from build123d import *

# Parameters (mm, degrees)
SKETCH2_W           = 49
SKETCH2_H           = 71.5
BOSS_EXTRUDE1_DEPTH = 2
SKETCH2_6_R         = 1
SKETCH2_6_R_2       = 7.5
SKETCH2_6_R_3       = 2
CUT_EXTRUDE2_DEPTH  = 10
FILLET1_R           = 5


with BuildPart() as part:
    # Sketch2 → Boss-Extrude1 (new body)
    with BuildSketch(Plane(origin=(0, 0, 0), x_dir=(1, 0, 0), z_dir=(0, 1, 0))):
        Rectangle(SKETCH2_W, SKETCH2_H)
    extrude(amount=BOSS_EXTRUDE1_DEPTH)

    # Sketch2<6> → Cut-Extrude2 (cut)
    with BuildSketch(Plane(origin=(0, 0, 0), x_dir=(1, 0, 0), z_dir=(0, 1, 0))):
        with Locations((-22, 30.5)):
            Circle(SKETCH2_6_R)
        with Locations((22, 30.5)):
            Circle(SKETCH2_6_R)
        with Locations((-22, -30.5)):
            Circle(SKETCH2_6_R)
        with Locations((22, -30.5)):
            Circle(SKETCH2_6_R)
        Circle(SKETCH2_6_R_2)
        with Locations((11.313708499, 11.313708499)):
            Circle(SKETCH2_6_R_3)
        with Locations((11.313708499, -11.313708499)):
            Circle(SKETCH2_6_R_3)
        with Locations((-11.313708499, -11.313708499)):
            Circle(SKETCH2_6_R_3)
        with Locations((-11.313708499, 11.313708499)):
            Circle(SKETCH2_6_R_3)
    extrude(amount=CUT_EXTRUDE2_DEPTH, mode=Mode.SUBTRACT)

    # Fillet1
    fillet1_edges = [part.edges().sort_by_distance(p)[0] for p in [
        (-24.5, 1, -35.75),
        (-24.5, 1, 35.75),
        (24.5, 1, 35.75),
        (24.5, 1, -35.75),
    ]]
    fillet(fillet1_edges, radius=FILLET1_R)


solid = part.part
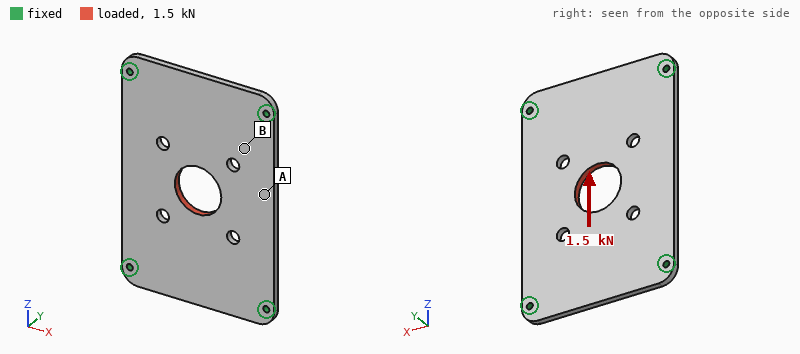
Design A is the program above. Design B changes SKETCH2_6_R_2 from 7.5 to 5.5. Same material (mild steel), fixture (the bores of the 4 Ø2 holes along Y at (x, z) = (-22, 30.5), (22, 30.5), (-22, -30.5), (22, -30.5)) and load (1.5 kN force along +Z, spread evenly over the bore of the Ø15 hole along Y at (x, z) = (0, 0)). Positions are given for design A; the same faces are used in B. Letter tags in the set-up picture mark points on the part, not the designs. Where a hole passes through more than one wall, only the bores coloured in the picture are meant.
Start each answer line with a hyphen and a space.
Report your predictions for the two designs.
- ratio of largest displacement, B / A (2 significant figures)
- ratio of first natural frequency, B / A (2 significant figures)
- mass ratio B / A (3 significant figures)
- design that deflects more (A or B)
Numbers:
- 1.1
- 0.99
- 1.03
- B
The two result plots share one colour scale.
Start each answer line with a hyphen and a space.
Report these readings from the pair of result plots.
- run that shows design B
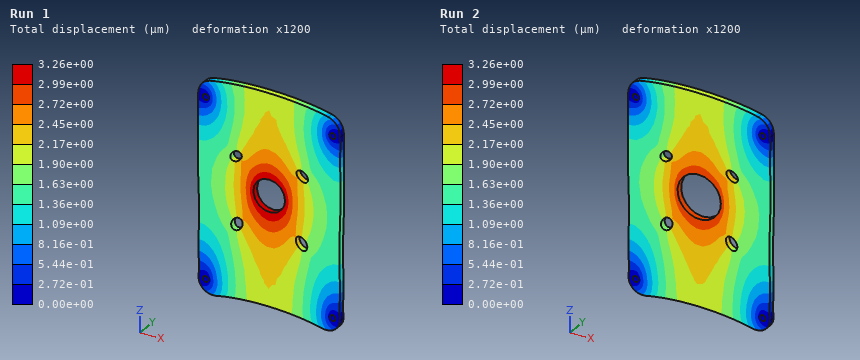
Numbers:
- Run 1
